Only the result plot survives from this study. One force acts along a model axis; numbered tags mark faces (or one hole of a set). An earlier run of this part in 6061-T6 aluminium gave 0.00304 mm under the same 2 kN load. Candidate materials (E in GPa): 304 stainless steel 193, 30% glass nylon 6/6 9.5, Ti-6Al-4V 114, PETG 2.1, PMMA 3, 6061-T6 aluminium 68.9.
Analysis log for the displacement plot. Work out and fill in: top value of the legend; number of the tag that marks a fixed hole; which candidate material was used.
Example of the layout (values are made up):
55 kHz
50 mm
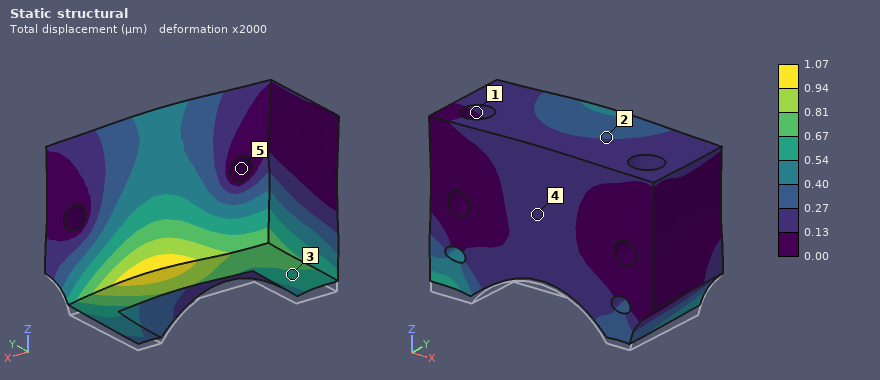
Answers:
1.07 µm
5
304 stainless steel
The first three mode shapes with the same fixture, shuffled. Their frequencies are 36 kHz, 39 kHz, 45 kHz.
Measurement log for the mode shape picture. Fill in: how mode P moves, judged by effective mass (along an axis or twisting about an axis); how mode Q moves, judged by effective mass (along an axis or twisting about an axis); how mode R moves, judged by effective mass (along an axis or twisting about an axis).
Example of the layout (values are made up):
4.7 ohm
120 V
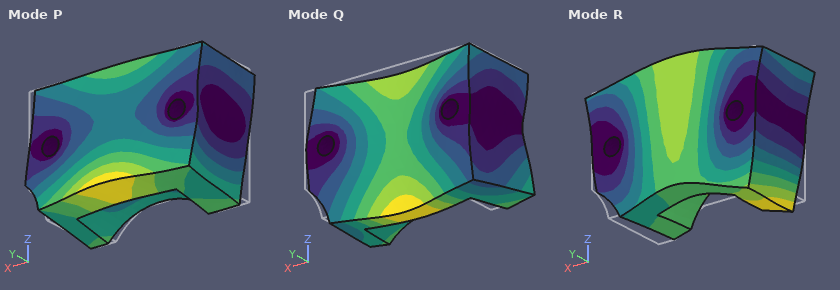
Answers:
twisting about X
along Y
along Z
